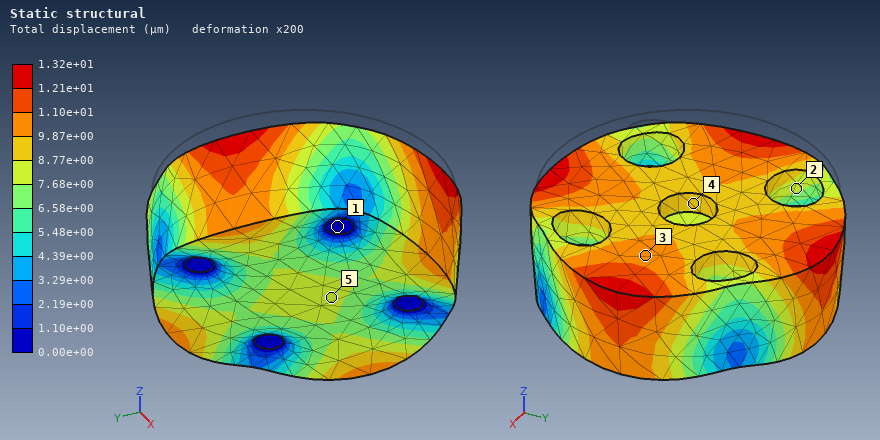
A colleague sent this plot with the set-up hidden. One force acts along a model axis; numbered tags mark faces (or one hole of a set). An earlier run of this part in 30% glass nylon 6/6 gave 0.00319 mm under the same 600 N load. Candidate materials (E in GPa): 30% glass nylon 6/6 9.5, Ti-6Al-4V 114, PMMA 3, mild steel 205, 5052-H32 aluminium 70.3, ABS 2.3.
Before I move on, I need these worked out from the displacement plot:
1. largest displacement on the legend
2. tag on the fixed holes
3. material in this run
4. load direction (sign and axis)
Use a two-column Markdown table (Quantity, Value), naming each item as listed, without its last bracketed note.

| Quantity | Value |
|---|---|
| largest displacement on the legend | 1.32e+01 µm |
| tag on the fixed holes | 1 |
| material in this run | ABS |
| load direction | -Z |
